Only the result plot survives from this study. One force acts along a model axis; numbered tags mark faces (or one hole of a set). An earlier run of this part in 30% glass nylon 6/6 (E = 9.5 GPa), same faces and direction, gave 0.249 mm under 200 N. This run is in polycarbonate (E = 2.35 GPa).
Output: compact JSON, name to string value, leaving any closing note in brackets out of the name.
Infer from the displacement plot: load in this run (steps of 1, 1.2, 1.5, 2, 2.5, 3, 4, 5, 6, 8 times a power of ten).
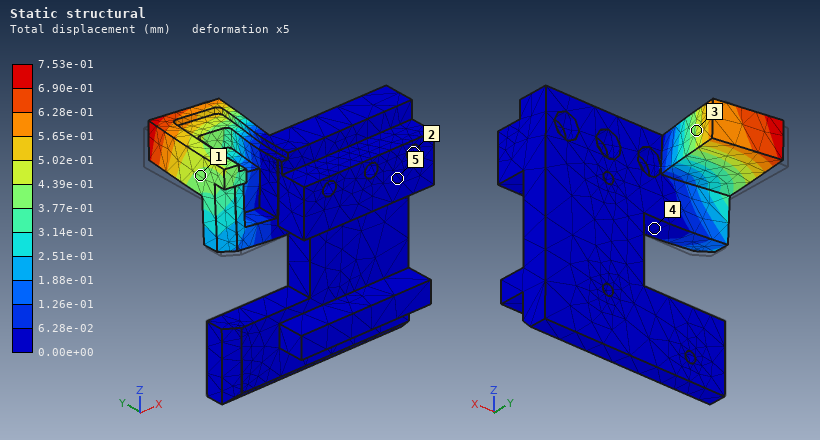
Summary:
{"load in this run": "150 N"}
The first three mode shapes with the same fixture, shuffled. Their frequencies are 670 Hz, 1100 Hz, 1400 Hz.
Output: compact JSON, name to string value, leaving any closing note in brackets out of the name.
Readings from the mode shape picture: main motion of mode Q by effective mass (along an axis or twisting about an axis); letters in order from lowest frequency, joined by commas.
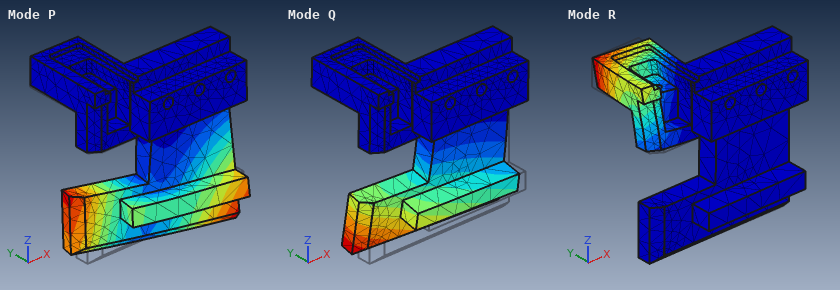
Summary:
{"main motion of mode Q by effective mass": "along Y", "letters in order from lowest frequency, joined by commas": "Q, R, P"}
